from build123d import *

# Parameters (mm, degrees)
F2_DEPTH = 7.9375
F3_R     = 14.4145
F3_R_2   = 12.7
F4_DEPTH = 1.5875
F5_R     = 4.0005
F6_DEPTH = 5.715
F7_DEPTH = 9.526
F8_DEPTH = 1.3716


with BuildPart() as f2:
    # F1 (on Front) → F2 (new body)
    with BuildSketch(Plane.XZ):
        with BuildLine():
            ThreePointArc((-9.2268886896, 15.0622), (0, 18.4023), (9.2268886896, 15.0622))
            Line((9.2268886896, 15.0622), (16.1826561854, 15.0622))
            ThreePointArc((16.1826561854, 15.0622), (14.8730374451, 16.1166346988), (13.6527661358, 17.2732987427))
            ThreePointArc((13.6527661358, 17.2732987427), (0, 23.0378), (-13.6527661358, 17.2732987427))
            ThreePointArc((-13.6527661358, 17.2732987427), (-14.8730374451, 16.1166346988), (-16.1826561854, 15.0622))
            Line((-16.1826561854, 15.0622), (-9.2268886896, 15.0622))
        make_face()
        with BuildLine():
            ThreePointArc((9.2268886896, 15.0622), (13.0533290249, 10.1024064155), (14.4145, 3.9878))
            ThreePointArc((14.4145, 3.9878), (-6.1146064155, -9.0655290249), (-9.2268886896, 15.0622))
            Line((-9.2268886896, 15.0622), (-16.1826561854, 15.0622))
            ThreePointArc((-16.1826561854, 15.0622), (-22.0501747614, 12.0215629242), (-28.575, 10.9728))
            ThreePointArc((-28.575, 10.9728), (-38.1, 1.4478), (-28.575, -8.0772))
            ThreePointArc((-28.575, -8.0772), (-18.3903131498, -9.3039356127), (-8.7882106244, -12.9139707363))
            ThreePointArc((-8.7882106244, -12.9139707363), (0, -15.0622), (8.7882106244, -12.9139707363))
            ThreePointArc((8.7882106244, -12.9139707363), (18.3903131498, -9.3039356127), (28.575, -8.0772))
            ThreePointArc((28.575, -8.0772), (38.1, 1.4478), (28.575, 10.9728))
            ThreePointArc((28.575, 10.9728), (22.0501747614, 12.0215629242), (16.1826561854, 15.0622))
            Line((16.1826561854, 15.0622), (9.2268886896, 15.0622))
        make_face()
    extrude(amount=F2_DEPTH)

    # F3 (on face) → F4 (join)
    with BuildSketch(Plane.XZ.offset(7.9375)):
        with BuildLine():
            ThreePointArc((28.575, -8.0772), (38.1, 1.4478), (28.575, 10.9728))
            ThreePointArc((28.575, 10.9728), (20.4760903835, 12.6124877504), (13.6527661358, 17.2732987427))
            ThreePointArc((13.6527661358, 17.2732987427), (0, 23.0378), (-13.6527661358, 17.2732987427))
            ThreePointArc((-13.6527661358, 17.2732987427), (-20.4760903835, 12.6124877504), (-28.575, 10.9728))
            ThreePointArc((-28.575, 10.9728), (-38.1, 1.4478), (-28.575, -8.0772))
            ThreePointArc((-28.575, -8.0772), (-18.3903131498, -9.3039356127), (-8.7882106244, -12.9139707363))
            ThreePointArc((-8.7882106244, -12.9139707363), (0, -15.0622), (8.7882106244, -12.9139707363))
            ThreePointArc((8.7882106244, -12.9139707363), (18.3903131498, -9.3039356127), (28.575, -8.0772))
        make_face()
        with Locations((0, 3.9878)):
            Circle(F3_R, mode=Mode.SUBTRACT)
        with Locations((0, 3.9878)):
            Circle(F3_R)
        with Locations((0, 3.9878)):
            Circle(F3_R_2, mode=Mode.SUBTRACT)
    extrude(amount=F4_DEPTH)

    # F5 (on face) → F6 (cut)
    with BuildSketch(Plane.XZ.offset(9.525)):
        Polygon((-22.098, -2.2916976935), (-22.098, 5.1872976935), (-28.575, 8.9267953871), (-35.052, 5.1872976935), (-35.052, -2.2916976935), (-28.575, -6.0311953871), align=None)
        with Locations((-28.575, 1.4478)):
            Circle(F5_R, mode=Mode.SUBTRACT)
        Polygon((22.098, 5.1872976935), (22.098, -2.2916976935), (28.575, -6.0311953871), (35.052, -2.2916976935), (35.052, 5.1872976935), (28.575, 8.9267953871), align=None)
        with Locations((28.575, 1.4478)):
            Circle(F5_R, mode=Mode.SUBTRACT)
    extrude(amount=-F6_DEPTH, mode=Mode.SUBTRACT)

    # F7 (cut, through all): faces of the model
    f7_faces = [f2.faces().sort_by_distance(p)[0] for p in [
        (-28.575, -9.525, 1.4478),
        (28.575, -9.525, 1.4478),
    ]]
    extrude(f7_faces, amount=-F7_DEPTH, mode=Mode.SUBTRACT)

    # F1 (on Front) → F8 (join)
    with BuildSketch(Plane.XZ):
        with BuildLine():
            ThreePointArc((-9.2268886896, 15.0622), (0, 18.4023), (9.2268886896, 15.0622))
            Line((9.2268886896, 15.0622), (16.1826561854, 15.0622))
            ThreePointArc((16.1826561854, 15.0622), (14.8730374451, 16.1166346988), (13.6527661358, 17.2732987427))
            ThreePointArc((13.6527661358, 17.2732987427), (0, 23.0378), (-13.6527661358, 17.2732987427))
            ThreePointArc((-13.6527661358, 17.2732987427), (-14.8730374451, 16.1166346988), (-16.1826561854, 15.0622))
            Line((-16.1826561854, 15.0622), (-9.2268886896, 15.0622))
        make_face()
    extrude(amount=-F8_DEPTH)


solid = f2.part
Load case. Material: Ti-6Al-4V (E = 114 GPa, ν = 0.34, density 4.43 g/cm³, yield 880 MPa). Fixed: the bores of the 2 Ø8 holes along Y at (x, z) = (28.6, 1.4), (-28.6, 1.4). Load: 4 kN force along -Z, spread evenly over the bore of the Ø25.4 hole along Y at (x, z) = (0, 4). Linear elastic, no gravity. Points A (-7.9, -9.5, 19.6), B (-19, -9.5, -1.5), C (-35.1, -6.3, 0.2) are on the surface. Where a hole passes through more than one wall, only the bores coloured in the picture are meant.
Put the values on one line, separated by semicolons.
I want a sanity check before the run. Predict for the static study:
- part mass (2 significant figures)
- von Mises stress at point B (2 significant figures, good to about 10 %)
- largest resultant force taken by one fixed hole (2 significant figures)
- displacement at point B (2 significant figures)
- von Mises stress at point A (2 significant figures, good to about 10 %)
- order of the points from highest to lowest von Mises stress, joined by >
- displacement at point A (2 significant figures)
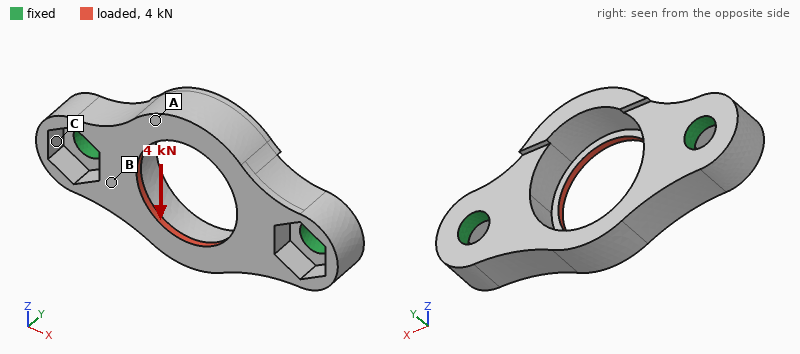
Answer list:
45 g; 67 MPa; 2.0 kN; 19 µm; 38 MPa; B > A > C; 53 µm
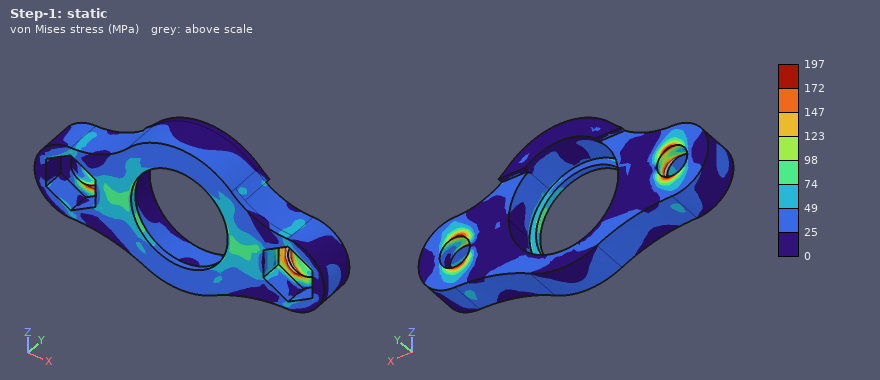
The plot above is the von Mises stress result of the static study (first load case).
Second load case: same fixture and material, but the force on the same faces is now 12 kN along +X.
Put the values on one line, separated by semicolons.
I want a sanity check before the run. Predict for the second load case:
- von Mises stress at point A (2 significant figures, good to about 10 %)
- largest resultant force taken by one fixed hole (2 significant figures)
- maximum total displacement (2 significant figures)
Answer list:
50 MPa; 6.1 kN; 36 µm
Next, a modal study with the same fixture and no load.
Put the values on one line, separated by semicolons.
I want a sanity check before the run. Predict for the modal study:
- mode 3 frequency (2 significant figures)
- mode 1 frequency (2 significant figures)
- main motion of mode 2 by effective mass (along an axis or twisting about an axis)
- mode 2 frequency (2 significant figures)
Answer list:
18 kHz; 7400 Hz; along Y; 9800 Hz
